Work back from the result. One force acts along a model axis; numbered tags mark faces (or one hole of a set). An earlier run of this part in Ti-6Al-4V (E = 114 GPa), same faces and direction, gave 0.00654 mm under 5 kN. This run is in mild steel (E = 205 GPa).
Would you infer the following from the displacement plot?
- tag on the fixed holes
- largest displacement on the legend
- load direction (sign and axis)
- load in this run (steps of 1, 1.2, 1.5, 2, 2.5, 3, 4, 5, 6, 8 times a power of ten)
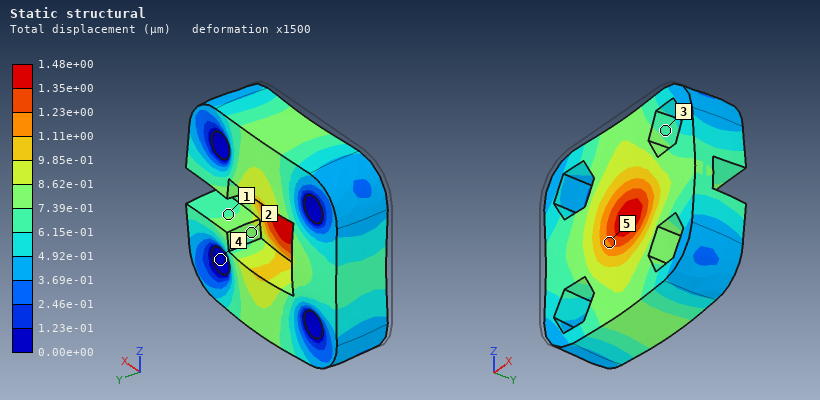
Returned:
4
1.48e+00 µm
+Y
2 kN
